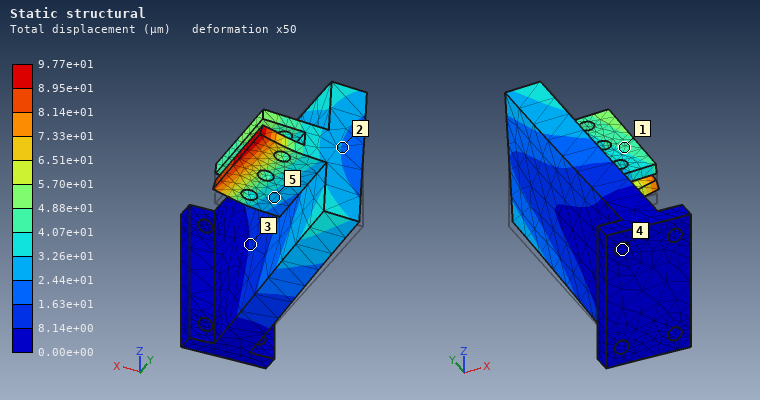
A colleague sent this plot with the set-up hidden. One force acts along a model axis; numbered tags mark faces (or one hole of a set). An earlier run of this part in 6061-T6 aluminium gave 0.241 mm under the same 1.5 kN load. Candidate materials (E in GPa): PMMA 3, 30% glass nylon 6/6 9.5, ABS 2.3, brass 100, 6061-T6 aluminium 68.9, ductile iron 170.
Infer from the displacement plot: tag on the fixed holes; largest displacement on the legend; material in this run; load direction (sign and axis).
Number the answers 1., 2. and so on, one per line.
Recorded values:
1. 4
2. 9.77e+01 µm
3. ductile iron
4. +Z
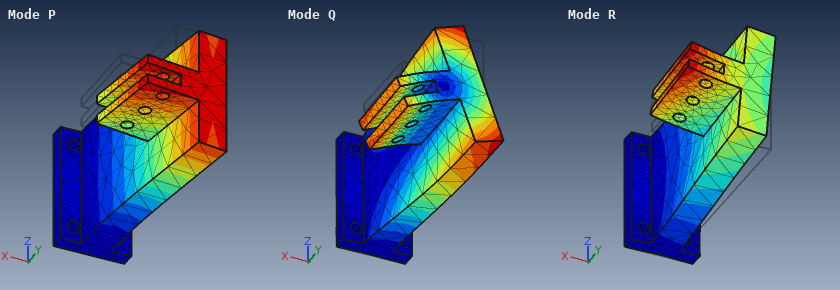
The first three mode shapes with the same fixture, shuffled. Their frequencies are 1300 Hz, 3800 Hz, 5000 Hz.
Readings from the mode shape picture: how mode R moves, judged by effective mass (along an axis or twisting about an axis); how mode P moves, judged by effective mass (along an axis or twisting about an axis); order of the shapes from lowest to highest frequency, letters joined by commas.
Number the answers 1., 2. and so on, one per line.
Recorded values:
1. along Z
2. along X
3. P, R, Q
